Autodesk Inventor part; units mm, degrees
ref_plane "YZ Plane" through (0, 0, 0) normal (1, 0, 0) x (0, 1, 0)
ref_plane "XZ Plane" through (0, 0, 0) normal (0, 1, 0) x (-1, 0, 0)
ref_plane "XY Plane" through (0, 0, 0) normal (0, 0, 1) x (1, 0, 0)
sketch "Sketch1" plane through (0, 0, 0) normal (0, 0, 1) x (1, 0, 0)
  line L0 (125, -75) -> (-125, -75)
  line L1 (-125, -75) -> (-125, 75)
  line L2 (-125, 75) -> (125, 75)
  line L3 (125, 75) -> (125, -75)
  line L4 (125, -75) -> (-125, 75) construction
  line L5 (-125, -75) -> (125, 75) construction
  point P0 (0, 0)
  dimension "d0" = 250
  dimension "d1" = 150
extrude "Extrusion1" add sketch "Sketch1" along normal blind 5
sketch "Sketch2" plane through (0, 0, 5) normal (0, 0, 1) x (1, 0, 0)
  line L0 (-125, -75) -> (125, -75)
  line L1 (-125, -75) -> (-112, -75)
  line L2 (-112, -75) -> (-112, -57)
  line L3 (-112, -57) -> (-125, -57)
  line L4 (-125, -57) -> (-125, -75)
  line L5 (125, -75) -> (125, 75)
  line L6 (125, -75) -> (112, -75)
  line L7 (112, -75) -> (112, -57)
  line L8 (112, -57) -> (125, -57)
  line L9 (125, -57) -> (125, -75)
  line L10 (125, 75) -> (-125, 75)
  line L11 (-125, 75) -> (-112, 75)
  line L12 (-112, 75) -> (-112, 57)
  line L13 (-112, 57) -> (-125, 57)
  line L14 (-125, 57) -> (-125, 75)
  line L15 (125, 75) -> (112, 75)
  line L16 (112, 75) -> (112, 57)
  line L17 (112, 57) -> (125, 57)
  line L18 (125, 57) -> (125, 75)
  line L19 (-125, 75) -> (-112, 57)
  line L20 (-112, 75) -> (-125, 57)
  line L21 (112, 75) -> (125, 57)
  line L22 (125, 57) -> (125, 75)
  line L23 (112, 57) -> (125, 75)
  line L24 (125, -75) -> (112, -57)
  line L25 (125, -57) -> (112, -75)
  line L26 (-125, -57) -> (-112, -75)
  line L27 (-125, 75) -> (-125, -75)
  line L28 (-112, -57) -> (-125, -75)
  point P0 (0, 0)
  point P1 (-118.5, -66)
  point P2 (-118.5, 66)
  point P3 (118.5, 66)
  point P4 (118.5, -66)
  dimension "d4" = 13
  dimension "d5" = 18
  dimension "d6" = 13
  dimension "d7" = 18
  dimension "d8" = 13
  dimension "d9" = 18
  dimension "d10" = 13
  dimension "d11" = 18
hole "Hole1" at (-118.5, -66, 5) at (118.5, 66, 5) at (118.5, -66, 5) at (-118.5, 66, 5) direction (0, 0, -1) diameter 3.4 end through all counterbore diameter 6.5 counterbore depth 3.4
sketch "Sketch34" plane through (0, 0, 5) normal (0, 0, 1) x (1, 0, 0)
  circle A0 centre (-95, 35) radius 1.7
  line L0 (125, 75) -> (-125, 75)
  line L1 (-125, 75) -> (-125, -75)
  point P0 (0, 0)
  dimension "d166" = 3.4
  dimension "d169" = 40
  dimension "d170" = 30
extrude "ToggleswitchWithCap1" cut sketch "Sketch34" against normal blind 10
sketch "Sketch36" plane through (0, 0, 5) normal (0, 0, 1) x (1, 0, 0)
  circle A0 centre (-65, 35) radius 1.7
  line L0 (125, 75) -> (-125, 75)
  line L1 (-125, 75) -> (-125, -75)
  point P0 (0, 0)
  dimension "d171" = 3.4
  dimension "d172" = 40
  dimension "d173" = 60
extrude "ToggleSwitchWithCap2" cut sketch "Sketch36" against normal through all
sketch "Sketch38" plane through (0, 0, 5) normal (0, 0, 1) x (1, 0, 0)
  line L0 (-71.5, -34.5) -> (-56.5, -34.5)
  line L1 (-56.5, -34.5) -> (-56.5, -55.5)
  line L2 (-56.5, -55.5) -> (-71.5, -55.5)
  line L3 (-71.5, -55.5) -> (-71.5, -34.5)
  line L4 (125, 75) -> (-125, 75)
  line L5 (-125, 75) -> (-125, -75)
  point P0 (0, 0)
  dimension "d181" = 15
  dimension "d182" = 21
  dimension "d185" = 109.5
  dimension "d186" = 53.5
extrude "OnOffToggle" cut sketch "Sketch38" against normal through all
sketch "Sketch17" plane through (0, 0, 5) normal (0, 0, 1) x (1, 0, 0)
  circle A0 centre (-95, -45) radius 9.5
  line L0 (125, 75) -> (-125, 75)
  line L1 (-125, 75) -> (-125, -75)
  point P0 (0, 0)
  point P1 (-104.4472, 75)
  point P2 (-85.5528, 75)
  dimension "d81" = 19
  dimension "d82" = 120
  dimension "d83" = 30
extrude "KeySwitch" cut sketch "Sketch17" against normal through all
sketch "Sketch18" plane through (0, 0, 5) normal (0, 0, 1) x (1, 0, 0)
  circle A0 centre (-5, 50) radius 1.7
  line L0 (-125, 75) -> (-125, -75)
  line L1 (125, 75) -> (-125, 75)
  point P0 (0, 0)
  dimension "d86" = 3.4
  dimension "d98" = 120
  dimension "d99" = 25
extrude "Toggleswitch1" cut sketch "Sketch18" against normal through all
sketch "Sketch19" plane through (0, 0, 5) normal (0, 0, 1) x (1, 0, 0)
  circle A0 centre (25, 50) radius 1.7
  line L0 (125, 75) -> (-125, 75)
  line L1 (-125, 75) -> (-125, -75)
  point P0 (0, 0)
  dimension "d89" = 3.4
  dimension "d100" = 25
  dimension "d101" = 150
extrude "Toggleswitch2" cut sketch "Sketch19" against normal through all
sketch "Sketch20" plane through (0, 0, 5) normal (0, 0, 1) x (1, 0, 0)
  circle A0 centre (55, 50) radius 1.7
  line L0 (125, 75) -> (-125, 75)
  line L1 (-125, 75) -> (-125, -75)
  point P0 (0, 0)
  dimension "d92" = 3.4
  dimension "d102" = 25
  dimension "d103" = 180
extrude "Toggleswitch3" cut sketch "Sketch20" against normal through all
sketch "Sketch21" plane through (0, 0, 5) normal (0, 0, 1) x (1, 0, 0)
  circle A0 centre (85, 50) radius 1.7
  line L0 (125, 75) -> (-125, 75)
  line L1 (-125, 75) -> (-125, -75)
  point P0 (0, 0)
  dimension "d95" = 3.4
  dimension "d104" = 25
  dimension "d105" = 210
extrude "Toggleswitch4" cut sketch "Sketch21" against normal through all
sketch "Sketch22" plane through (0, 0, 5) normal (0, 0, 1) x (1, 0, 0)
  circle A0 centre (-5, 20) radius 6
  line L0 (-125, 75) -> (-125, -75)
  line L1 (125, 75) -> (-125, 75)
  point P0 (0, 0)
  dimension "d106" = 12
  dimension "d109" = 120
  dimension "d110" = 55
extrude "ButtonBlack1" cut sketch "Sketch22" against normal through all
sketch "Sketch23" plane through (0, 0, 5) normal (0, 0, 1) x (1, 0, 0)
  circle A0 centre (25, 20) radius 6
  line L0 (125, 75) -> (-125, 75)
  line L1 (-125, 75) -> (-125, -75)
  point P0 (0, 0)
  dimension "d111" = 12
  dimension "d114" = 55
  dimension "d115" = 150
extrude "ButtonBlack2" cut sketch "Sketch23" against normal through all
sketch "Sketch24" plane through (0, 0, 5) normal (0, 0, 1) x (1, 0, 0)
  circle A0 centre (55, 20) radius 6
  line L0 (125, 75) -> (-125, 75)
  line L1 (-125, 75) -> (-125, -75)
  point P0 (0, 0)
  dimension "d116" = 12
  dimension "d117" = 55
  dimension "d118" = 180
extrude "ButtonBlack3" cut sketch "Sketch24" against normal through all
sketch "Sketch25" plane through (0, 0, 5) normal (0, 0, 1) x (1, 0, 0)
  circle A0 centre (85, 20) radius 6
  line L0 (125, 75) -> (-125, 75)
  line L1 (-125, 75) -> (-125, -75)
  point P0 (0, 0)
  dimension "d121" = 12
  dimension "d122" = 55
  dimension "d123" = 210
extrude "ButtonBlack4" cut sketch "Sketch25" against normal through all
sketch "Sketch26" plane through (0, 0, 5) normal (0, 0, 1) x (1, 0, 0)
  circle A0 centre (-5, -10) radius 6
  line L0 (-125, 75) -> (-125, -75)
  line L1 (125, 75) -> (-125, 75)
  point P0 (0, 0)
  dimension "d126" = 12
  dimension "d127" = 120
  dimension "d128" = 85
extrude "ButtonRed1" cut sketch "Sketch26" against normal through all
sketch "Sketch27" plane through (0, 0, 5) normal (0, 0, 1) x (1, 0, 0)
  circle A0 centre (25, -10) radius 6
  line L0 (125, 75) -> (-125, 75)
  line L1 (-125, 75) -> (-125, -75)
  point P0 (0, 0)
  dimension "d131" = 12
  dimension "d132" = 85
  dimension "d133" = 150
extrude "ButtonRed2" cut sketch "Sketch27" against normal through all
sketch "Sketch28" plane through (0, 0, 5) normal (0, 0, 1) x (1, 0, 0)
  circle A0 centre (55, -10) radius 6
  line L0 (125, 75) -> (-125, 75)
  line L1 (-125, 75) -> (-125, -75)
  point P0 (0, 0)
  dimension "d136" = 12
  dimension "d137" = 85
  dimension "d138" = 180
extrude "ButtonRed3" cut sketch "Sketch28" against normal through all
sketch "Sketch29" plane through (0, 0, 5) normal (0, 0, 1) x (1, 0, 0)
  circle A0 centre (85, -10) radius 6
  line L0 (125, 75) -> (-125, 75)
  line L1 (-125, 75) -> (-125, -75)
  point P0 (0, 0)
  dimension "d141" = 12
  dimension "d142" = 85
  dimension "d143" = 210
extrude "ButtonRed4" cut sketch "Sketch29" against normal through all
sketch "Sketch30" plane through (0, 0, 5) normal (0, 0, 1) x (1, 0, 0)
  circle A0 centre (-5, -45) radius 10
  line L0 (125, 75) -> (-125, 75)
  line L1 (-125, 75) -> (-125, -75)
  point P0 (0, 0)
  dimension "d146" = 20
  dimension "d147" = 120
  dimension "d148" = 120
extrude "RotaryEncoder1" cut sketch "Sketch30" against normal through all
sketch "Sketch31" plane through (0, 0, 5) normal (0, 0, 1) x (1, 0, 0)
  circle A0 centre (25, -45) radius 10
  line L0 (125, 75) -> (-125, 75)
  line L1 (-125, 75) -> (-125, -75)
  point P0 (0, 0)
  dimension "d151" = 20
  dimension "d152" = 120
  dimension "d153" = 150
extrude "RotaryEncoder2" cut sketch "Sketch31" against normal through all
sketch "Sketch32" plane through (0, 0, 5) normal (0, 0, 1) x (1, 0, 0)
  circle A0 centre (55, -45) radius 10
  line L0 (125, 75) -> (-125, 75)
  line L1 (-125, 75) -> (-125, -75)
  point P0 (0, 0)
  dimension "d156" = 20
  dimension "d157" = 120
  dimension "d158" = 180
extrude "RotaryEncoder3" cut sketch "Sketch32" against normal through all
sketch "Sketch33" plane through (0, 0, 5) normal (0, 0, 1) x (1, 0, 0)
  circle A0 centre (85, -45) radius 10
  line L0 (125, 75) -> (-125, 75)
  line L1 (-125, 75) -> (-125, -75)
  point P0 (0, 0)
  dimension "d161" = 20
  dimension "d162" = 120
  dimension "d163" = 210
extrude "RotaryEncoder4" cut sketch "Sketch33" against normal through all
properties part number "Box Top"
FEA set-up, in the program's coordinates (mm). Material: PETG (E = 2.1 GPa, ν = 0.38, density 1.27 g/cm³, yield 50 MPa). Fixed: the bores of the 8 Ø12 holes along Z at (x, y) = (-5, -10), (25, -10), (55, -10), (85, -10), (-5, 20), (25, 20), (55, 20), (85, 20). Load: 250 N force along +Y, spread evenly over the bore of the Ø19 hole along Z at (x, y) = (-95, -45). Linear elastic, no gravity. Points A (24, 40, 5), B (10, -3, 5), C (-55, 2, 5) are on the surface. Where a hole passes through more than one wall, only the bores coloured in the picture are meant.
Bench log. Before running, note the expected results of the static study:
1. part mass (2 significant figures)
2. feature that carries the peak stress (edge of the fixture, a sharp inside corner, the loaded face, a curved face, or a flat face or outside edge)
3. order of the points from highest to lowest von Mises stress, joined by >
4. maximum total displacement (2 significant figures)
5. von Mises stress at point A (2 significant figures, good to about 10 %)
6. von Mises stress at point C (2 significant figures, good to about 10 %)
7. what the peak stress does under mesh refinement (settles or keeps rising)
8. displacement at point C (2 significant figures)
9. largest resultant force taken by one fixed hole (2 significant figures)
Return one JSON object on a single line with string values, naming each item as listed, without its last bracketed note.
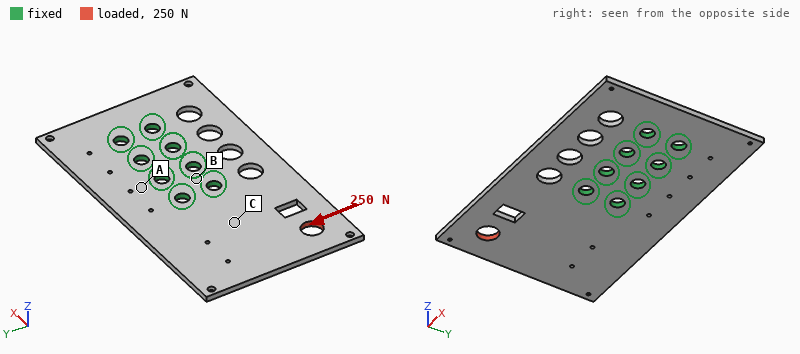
{"part mass": "220 g", "feature that carries the peak stress": "edge of the fixture", "order of the points from highest to lowest von Mises stress, joined by >": "C > A > B", "maximum total displacement": "0.19 mm", "von Mises stress at point A": "0.67 MPa", "von Mises stress at point C": "0.98 MPa", "what the peak stress does under mesh refinement": "keeps rising", "displacement at point C": "0.066 mm", "largest resultant force taken by one fixed hole": "250 N"}
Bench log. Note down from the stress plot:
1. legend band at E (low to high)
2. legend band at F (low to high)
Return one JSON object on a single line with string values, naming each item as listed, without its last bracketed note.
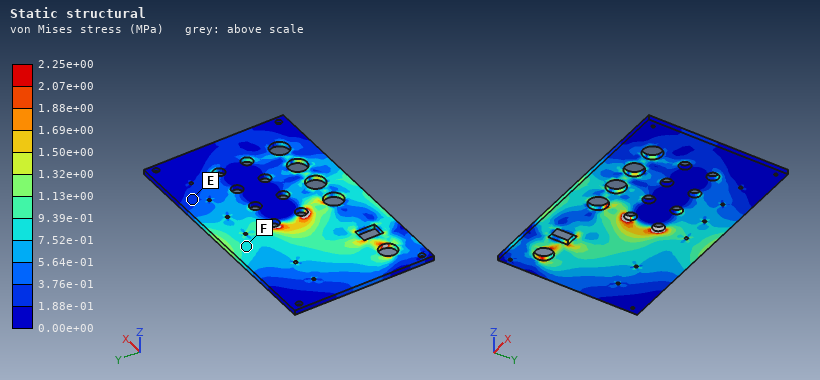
{"legend band at E": "1.88e-01 to 3.76e-01 MPa", "legend band at F": "7.52e-01 to 9.39e-01 MPa"}
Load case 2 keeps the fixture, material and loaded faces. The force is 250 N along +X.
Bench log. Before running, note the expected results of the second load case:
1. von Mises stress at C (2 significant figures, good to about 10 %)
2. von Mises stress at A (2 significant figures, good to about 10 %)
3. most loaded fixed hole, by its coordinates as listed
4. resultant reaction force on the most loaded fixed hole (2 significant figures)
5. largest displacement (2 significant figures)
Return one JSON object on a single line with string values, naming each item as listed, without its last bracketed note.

{"von Mises stress at C": "0.43 MPa", "von Mises stress at A": "0.21 MPa", "most loaded fixed hole, by its coordinates as listed": "(-5, -10)", "resultant reaction force on the most loaded fixed hole": "180 N", "largest displacement": "0.11 mm"}
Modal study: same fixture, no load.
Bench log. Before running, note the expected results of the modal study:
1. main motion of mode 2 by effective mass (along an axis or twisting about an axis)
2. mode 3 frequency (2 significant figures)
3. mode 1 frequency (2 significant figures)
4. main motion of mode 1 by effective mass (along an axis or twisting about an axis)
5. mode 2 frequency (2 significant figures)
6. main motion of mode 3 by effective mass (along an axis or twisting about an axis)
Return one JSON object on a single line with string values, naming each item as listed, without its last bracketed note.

{"main motion of mode 2 by effective mass": "twisting about X", "mode 3 frequency": "260 Hz", "mode 1 frequency": "73 Hz", "main motion of mode 1 by effective mass": "along Z", "mode 2 frequency": "120 Hz", "main motion of mode 3 by effective mass": "along Z"}
